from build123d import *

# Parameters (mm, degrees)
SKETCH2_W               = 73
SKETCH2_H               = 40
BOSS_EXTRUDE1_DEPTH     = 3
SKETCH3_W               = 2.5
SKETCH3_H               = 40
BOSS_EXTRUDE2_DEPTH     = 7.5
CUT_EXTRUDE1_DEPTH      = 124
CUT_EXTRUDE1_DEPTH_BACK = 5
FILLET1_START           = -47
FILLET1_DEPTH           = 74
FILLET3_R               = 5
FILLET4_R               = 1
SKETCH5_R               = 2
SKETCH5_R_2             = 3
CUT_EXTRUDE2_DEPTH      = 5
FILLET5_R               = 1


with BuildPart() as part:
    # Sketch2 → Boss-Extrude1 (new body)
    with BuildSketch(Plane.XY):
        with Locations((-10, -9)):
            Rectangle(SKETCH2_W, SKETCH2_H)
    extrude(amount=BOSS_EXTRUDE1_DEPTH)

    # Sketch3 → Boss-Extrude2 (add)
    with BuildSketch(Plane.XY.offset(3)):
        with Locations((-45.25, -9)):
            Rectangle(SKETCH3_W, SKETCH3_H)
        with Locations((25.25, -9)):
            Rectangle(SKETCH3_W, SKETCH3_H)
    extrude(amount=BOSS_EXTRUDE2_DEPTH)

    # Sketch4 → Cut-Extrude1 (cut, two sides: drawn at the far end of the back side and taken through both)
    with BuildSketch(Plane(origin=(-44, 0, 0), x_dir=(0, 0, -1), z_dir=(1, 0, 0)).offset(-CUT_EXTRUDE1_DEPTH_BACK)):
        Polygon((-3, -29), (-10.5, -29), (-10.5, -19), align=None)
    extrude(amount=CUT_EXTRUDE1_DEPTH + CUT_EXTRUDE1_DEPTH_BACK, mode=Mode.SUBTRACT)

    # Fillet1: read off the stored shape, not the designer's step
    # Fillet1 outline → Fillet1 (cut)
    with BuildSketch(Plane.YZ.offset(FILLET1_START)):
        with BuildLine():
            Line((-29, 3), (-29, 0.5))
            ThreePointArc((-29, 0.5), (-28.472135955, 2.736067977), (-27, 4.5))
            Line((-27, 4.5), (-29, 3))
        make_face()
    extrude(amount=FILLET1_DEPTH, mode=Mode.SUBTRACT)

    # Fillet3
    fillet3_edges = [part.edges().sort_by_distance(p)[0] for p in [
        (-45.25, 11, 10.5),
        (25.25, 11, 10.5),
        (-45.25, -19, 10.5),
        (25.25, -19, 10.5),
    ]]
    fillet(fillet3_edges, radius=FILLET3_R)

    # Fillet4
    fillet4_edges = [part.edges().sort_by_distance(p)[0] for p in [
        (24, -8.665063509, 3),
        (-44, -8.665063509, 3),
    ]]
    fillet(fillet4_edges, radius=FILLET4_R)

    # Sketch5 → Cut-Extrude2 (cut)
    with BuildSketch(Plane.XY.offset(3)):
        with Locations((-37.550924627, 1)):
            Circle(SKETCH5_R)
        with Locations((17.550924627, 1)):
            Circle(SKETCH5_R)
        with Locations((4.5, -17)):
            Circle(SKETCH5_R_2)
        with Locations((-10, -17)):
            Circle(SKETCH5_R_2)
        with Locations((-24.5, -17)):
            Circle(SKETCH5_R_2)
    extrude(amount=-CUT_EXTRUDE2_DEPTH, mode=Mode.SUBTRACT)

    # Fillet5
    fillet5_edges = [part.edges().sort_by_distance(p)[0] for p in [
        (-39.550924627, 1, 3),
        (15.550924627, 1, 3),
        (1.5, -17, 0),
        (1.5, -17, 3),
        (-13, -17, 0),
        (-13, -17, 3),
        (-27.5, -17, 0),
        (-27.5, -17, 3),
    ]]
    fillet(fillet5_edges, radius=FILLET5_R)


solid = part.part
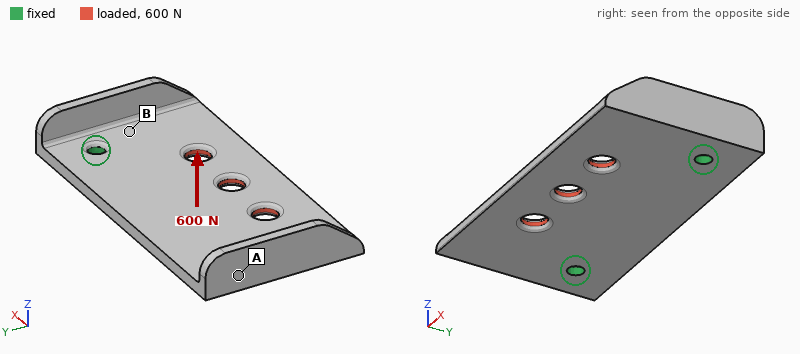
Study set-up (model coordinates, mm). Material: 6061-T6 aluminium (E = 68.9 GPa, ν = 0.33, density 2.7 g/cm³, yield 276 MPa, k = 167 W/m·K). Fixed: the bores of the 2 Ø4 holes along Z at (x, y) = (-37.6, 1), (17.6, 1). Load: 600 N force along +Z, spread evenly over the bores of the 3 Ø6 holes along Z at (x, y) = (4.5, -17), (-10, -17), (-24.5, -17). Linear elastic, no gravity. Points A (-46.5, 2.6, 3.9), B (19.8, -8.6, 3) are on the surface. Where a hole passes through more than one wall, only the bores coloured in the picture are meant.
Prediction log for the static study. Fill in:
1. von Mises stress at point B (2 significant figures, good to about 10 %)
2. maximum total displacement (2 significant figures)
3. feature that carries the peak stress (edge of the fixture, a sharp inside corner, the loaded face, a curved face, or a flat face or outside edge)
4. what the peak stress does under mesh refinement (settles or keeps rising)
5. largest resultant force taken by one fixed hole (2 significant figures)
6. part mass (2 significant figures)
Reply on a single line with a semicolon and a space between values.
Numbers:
61 MPa; 0.40 mm; edge of the fixture; keeps rising; 310 N; 26 g
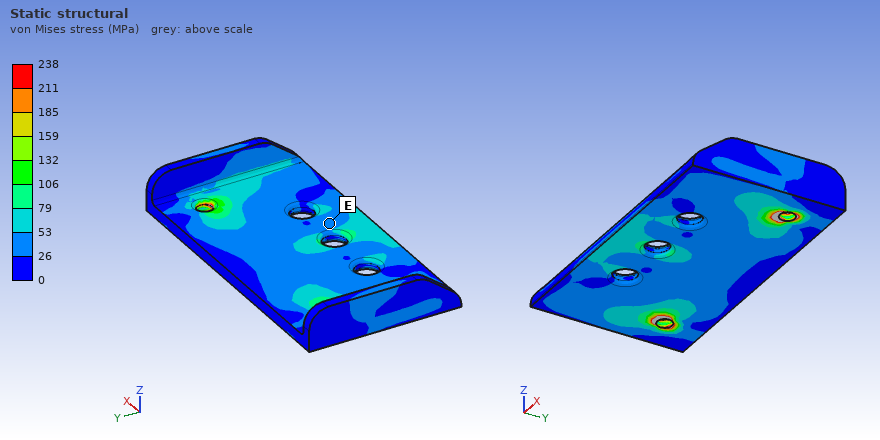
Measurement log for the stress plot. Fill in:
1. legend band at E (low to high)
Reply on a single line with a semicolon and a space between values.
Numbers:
26 to 53 MPa
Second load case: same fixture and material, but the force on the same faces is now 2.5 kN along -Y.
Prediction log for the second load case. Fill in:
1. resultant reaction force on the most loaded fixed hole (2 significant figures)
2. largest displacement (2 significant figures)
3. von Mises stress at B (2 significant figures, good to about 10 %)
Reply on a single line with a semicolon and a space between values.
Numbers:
1.3 kN; 19 µm; 14 MPa
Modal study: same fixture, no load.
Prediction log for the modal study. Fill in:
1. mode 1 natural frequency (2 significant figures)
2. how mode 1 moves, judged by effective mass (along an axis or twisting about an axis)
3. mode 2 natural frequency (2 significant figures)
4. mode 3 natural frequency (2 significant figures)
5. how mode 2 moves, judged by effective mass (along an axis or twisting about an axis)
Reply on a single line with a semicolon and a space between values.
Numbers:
2400 Hz; along Z; 3800 Hz; 4400 Hz; twisting about Y
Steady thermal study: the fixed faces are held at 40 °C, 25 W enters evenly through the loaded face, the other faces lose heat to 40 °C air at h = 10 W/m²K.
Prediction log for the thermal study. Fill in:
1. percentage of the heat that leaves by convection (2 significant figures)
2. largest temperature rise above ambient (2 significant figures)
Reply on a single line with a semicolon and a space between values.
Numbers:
3.5 %; 27 K
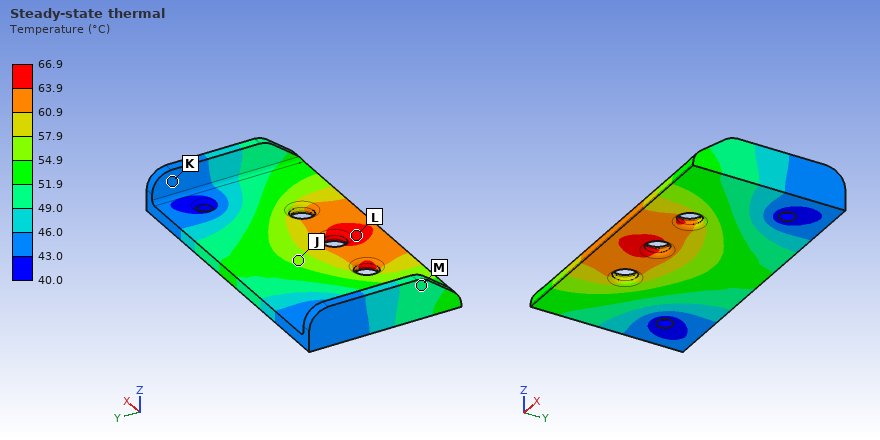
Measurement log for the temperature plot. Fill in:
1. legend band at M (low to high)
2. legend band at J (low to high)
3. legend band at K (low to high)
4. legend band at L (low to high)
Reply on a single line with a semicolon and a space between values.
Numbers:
49.0 to 51.9 °C; 54.9 to 57.9 °C; 43.0 to 46.0 °C; 63.9 to 66.9 °C
